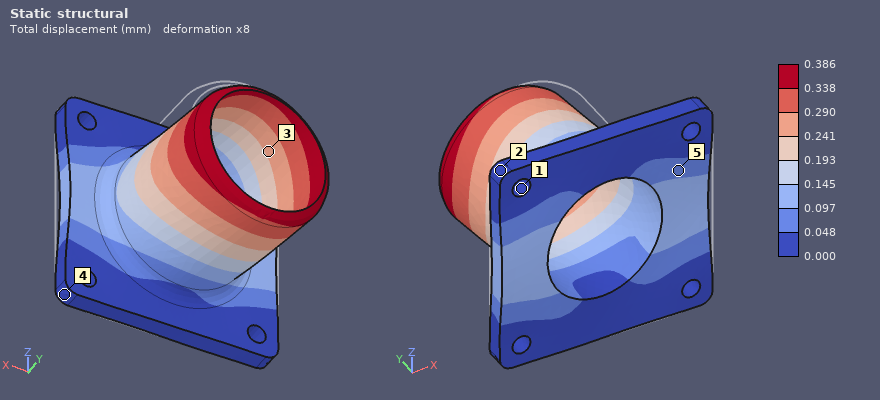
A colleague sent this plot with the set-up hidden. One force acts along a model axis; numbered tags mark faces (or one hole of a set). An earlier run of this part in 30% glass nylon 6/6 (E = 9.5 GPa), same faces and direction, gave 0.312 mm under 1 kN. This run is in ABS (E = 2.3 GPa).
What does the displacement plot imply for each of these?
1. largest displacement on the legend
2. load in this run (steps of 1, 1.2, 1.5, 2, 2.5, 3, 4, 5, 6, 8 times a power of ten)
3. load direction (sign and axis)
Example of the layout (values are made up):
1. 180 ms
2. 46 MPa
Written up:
1. 0.386 mm
2. 300 N
3. -X
